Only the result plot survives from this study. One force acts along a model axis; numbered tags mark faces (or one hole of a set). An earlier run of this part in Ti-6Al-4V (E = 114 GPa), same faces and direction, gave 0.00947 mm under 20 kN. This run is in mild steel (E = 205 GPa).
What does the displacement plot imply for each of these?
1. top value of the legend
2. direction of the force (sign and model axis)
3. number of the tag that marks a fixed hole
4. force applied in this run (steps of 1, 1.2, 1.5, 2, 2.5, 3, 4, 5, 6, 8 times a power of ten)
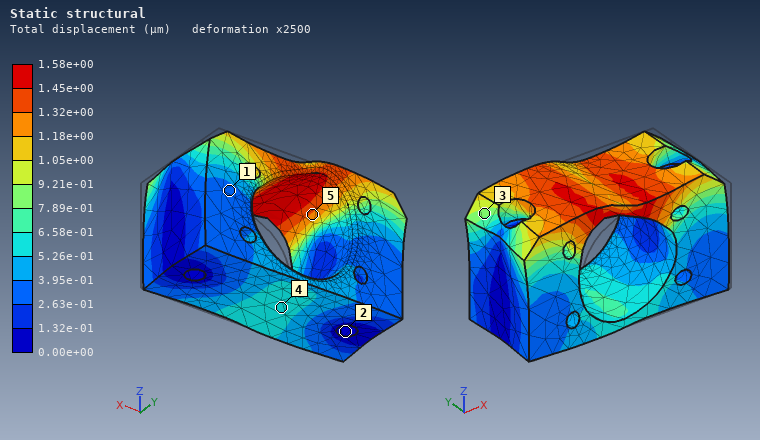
1.58e+00 µm
-X
2
6 kN
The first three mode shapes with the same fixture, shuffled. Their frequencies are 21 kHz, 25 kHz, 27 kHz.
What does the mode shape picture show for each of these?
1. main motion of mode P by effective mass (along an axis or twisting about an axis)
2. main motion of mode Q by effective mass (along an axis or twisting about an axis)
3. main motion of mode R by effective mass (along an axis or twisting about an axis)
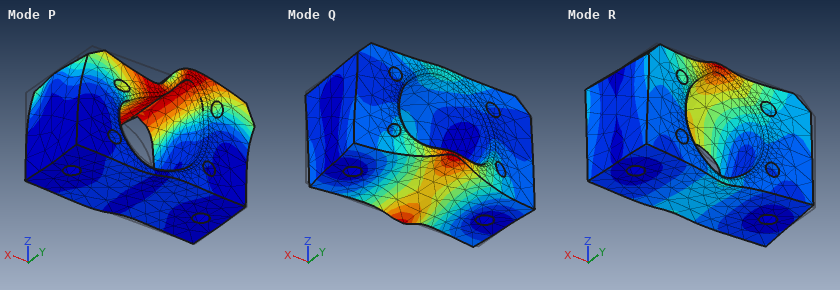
along X
twisting about X
along Y
